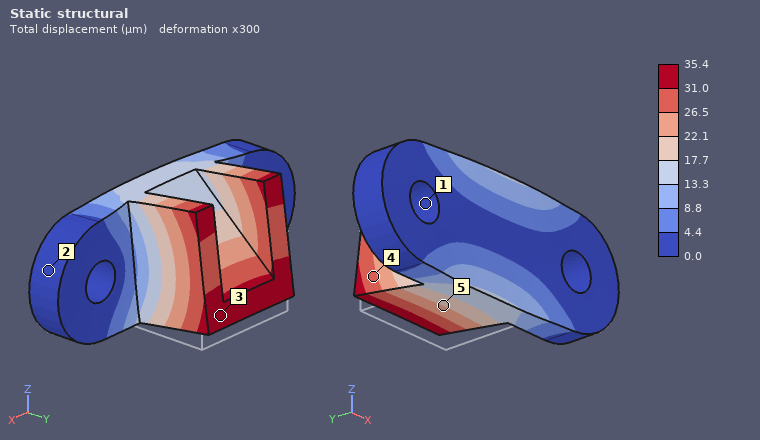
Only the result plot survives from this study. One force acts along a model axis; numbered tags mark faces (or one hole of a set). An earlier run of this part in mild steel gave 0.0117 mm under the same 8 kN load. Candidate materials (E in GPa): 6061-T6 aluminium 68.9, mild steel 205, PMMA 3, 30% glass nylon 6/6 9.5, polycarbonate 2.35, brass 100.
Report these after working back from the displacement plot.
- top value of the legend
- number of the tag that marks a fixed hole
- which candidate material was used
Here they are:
35.4 µm
1
6061-T6 aluminium
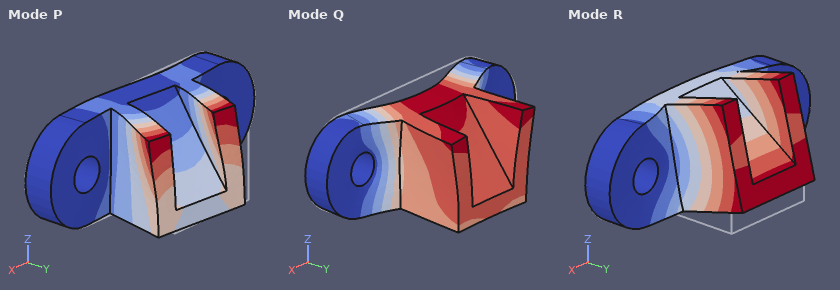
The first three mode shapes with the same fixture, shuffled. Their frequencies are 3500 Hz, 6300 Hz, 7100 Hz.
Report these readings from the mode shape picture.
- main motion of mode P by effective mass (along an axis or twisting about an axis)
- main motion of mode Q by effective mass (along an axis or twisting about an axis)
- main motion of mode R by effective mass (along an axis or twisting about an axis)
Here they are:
along X
along Y
along Z
